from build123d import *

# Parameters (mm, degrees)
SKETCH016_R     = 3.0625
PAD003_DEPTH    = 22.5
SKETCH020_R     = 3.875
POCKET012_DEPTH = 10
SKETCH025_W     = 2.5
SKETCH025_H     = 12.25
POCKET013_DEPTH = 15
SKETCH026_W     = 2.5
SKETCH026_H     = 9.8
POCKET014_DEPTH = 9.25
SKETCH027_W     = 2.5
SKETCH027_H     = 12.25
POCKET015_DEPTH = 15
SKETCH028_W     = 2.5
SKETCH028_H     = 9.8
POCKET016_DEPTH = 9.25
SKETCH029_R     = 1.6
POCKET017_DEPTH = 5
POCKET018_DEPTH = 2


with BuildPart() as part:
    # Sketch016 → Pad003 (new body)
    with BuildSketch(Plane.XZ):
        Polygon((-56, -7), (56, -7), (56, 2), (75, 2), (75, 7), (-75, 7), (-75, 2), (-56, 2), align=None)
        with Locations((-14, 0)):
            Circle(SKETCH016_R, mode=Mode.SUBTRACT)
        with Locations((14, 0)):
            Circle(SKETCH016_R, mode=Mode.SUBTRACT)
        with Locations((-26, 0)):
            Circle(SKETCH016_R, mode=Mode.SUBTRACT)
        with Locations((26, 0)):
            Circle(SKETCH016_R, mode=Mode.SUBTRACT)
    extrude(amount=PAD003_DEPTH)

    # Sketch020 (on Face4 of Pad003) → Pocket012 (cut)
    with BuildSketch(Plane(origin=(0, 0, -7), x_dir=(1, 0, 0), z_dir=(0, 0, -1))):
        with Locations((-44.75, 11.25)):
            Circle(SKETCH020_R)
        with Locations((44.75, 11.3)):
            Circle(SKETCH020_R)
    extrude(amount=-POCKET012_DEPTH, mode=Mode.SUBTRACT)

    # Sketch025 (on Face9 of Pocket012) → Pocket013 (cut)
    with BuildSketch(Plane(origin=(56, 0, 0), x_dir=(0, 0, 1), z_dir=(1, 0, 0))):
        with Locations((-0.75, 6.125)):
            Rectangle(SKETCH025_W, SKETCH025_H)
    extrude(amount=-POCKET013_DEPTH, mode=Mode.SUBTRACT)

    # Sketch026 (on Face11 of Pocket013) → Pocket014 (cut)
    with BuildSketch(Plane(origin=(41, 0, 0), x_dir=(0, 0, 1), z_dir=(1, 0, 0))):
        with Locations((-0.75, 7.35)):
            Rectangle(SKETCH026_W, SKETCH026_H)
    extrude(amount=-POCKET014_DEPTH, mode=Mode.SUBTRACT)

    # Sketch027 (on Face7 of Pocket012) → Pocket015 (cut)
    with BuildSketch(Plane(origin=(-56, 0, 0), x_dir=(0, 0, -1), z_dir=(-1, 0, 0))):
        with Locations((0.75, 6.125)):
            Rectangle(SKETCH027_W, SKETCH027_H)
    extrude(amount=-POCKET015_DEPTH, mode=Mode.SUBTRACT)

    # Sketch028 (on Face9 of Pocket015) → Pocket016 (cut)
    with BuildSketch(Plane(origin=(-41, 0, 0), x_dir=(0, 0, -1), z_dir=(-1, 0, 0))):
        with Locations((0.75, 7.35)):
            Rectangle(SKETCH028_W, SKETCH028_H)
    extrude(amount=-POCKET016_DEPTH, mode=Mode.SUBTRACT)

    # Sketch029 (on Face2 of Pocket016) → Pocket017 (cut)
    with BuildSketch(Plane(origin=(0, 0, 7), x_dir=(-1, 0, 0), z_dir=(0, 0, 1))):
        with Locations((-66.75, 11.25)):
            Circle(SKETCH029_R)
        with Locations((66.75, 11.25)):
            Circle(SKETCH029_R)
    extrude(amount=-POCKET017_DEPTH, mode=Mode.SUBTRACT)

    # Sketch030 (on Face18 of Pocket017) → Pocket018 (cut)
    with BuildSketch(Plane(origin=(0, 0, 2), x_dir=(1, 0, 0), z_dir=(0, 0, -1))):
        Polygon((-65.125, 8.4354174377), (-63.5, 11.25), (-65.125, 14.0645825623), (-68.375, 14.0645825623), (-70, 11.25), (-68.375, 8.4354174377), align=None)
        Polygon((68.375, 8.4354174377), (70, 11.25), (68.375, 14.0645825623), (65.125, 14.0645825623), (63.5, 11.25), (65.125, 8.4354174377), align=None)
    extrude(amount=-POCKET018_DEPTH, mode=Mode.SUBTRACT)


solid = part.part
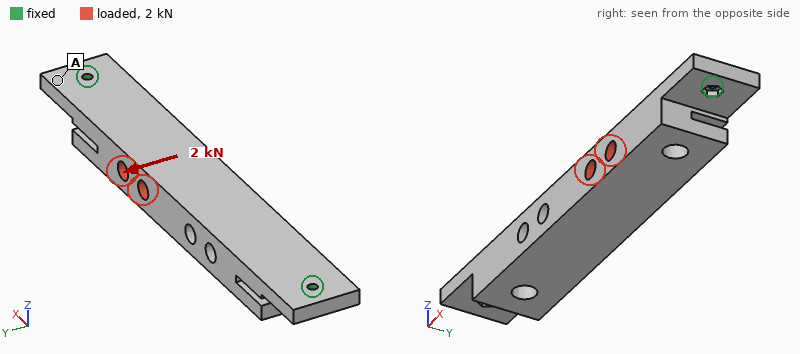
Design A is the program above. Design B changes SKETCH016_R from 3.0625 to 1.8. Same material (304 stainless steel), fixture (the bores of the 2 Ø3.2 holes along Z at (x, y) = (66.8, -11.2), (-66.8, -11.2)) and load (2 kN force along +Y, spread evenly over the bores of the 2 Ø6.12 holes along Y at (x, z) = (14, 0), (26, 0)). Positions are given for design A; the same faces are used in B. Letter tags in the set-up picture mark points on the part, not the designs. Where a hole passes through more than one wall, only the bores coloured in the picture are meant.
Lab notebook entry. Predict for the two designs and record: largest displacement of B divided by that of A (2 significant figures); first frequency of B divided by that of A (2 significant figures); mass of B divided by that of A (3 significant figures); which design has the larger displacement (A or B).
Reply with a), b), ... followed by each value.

a) 0.92
b) 1.00
c) 1.05
d) A
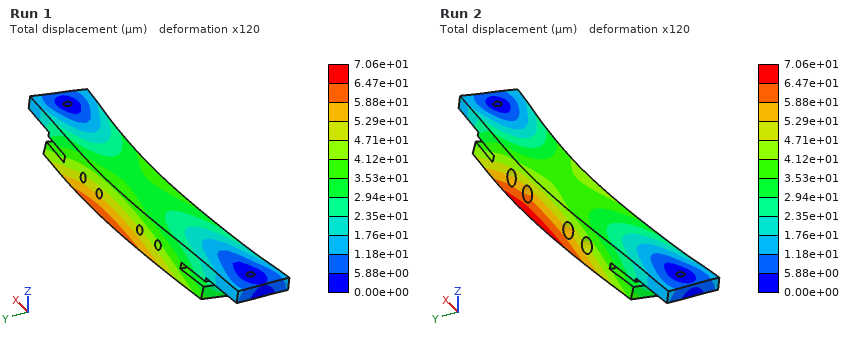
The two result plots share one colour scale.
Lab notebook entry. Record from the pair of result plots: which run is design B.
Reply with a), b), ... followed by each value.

a) Run 1
